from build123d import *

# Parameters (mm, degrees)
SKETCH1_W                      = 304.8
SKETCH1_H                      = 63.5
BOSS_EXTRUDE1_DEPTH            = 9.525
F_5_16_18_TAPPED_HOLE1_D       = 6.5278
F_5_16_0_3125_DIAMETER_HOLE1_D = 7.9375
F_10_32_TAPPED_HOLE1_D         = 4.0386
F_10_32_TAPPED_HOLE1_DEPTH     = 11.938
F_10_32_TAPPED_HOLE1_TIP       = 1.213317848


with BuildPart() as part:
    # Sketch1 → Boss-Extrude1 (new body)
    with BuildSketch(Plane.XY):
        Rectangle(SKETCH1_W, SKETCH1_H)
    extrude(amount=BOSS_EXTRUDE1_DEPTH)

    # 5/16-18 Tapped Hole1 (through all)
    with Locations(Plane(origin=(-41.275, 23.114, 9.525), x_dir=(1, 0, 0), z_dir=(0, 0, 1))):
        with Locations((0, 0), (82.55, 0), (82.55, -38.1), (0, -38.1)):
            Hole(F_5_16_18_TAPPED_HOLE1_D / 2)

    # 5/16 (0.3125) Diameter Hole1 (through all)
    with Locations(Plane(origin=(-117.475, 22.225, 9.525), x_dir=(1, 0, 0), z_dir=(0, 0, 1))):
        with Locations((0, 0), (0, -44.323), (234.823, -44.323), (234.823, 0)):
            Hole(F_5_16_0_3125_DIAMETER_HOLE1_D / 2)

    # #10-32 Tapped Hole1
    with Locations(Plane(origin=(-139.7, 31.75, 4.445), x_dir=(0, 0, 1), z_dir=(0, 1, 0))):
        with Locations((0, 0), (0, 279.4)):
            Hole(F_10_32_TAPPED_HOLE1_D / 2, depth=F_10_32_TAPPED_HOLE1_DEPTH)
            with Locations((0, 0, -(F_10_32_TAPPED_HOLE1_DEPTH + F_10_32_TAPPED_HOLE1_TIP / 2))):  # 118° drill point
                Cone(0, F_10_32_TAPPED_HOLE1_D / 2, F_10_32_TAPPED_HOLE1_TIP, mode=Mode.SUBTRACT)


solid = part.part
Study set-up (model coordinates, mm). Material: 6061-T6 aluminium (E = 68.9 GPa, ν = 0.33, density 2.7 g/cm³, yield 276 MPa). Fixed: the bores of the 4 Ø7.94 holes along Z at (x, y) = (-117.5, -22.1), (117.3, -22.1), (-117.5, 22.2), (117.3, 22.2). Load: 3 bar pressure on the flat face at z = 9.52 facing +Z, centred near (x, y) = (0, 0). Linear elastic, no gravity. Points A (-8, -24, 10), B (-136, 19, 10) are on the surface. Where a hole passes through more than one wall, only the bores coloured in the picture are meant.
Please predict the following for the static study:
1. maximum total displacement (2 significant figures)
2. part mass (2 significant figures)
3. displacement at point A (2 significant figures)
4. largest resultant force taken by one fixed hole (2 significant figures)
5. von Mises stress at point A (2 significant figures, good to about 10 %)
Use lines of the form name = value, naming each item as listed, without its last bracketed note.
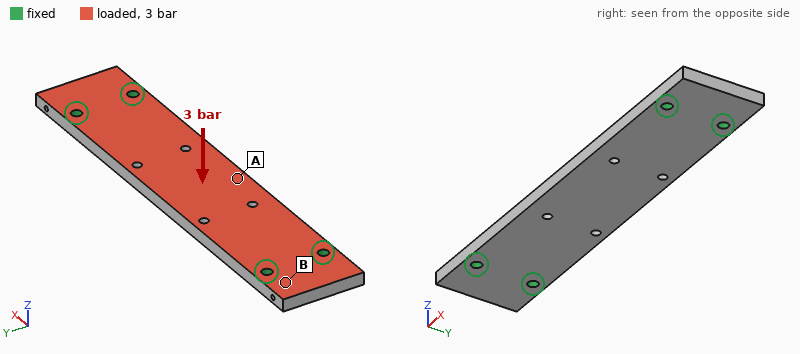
maximum total displacement = 0.49 mm
part mass = 490 g
displacement at point A = 0.47 mm
largest resultant force taken by one fixed hole = 1.4 kN
von Mises stress at point A = 44 MPa
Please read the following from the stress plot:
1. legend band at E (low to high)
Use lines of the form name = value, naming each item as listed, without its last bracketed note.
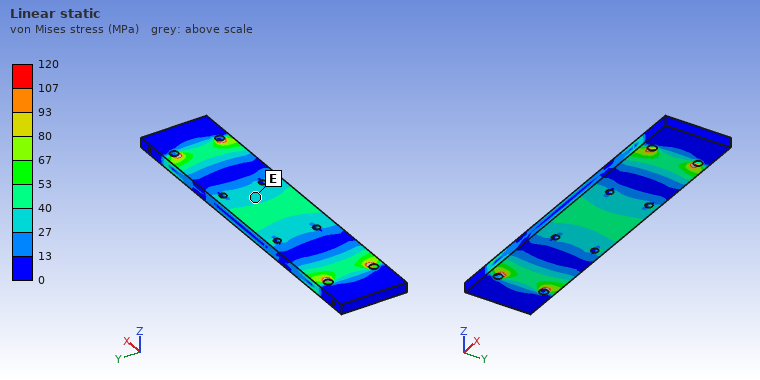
legend band at E = 27 to 40 MPa
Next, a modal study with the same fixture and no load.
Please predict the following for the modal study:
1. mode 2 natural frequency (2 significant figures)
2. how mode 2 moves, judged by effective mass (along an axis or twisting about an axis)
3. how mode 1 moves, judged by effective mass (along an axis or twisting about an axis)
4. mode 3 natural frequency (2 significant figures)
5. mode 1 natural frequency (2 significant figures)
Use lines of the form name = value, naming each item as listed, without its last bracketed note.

mode 2 natural frequency = 2200 Hz
how mode 2 moves, judged by effective mass = twisting about X
how mode 1 moves, judged by effective mass = along Z
mode 3 natural frequency = 2400 Hz
mode 1 natural frequency = 900 Hz
